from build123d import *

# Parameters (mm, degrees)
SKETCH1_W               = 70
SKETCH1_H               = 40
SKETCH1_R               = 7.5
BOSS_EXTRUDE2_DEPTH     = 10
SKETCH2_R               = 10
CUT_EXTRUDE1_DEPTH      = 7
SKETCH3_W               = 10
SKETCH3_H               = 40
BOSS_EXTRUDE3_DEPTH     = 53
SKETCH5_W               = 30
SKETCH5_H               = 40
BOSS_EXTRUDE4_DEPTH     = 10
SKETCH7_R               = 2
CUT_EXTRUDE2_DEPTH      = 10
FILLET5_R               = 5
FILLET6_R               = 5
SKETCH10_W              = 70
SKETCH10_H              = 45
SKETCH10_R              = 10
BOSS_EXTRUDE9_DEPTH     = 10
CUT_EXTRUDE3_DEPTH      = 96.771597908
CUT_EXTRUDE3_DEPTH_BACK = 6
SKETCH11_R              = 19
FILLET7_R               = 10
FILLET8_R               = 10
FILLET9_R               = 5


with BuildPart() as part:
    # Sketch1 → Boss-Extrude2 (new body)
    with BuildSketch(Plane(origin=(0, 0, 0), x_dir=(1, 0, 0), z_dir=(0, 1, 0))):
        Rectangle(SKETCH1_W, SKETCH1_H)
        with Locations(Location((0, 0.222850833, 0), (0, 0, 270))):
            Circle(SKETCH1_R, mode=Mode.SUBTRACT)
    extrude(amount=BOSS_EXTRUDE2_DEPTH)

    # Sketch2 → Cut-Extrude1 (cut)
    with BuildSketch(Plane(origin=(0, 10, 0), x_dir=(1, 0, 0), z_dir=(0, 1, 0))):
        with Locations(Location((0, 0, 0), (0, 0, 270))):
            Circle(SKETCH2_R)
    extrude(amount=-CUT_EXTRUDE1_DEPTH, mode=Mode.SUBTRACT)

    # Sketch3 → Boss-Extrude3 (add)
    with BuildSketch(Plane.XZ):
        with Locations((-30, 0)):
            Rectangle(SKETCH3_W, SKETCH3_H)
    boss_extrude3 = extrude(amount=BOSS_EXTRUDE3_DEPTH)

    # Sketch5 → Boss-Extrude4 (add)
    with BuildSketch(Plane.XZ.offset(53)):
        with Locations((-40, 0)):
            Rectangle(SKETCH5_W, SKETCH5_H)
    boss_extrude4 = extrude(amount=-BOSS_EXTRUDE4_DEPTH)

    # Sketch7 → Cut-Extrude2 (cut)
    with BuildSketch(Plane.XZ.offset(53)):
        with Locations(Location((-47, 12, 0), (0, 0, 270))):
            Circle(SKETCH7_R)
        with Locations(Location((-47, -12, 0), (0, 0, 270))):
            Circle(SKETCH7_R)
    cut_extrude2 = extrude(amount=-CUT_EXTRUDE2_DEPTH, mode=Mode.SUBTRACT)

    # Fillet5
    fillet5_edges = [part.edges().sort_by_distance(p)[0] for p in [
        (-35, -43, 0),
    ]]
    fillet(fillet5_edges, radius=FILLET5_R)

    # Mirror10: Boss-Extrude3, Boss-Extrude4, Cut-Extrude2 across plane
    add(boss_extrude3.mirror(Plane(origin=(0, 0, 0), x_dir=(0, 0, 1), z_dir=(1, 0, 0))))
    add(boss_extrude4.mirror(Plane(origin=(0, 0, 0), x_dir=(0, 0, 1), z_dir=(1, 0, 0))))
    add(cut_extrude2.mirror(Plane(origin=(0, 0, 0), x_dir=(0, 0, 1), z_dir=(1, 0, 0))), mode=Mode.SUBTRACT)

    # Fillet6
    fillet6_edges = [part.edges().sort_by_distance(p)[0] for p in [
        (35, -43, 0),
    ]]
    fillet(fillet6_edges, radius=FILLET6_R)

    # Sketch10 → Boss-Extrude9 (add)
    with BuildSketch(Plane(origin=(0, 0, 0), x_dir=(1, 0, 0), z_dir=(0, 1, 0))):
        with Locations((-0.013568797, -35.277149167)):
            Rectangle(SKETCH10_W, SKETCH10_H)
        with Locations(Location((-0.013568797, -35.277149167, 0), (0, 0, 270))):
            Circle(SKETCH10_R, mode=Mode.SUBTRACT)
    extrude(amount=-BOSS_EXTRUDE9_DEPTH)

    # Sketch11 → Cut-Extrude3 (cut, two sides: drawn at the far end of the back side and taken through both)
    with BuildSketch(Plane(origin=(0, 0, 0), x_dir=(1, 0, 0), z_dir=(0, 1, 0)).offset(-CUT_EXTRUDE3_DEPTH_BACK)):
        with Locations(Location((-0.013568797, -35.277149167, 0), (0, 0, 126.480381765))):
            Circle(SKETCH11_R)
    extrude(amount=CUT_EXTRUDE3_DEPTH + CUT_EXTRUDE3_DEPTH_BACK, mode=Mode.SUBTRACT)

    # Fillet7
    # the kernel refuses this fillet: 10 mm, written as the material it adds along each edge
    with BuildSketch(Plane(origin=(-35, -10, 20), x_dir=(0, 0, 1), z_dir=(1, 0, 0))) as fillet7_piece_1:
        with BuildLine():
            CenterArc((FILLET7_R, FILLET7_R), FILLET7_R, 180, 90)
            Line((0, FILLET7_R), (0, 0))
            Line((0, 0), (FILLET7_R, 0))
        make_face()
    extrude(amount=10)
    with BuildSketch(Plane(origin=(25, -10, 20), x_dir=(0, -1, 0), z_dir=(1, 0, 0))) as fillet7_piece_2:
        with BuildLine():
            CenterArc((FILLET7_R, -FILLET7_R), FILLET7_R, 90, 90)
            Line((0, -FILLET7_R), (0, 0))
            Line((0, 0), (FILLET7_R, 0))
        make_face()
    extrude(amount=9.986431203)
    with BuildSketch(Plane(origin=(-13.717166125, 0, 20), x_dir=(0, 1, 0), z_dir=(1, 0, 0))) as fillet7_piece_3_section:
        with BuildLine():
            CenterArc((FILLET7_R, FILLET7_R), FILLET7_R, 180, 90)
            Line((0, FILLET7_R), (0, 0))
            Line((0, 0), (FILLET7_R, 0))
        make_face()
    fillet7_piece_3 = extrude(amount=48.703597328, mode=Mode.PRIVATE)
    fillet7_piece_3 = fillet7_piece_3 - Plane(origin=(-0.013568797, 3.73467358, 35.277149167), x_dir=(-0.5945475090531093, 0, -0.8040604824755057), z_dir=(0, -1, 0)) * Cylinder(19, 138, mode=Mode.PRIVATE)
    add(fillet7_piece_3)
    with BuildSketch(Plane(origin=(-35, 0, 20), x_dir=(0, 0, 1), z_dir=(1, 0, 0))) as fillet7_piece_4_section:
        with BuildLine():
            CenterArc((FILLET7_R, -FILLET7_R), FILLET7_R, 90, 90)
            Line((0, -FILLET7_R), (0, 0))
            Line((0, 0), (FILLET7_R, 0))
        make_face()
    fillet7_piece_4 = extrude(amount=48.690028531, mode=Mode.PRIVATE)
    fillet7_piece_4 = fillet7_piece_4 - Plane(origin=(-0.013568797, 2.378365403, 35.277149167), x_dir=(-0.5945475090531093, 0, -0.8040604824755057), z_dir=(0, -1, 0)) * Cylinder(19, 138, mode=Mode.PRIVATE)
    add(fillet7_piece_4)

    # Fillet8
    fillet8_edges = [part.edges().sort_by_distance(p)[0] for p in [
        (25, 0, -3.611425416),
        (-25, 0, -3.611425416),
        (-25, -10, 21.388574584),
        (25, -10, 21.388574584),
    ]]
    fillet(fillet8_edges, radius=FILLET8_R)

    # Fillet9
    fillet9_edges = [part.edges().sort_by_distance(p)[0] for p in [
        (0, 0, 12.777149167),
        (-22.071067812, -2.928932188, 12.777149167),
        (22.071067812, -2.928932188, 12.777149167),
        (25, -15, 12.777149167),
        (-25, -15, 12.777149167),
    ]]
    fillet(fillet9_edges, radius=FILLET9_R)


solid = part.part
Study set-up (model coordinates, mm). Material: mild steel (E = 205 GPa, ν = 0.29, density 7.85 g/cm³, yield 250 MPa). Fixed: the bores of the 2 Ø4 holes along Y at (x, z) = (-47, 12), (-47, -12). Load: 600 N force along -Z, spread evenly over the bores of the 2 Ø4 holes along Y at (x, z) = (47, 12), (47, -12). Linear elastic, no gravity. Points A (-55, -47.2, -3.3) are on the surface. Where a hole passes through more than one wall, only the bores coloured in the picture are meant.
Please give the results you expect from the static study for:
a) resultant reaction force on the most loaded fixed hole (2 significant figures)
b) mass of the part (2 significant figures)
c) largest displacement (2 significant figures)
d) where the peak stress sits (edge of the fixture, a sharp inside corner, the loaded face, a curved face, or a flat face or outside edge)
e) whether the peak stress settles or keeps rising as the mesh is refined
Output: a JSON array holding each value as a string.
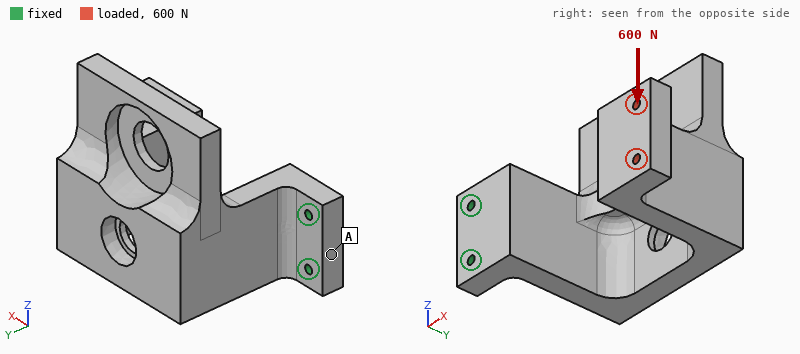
["2.2 kN", "850 g", "0.24 mm", "edge of the fixture", "keeps rising"]
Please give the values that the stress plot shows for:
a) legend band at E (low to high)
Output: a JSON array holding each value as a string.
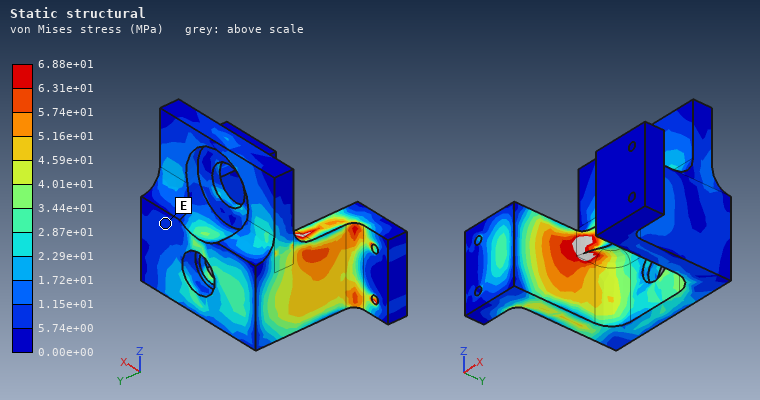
["5.74e+00 to 1.15e+01 MPa"]
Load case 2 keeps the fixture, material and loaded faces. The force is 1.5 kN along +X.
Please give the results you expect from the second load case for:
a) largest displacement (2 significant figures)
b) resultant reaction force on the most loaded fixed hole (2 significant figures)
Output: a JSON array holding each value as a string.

["0.43 mm", "750 N"]
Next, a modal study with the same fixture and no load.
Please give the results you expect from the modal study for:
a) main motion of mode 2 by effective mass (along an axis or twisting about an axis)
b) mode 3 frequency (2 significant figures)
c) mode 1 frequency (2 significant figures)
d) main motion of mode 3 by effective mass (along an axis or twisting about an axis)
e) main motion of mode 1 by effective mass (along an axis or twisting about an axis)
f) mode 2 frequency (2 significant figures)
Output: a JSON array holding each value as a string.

["along Z", "1100 Hz", "370 Hz", "along X", "along Y", "590 Hz"]
